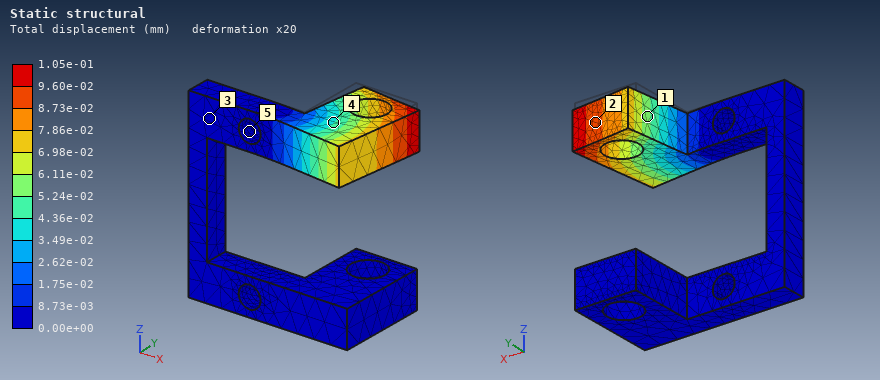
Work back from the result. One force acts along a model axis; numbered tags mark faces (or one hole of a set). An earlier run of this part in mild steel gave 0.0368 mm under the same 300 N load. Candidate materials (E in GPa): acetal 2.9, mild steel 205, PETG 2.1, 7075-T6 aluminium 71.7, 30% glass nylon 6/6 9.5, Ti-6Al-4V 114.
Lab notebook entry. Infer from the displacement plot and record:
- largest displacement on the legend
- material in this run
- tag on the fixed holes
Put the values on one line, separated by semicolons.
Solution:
1.05e-01 mm; 7075-T6 aluminium; 5
